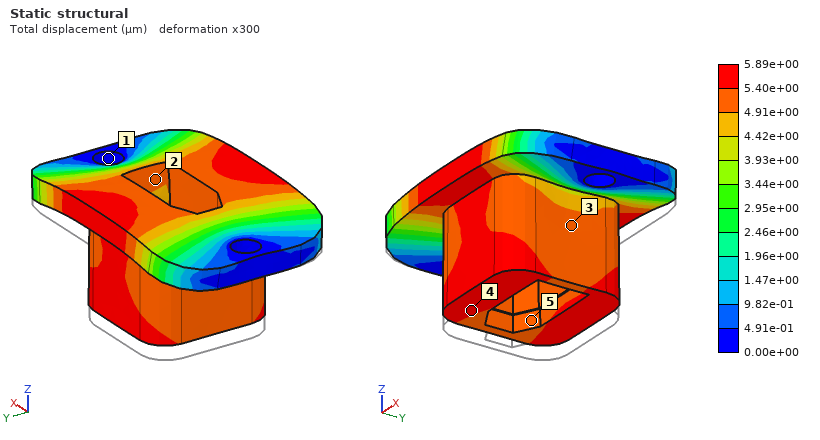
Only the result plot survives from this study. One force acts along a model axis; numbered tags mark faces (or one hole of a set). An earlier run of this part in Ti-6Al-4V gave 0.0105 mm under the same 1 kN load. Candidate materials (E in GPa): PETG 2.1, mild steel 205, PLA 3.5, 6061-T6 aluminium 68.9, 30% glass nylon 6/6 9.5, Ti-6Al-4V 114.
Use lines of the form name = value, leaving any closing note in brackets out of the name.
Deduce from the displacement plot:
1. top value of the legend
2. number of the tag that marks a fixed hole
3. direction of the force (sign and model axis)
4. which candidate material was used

top value of the legend = 5.89e+00 µm
number of the tag that marks a fixed hole = 1
direction of the force = +Z
which candidate material was used = mild steel
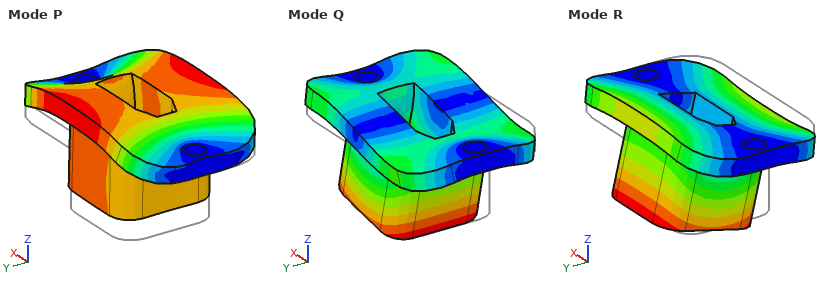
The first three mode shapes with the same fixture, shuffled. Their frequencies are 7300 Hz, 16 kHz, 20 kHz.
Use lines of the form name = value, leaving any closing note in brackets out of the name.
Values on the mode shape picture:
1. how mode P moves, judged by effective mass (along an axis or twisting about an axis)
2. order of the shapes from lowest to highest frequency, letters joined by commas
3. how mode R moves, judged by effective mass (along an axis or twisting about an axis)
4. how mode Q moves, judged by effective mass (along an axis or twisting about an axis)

how mode P moves, judged by effective mass = along Z
order of the shapes from lowest to highest frequency, letters joined by commas = R, P, Q
how mode R moves, judged by effective mass = along Y
how mode Q moves, judged by effective mass = along X
